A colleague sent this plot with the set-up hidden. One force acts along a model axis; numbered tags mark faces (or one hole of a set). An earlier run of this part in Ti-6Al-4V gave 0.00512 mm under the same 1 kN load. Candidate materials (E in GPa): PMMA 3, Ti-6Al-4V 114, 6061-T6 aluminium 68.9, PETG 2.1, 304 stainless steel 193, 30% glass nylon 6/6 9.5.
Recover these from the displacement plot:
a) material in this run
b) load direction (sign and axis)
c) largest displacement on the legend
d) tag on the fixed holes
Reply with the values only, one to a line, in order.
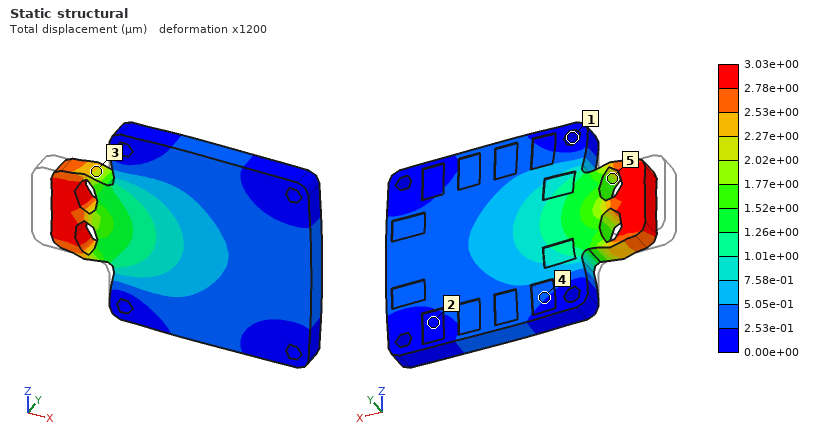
304 stainless steel
+X
3.03e+00 µm
1
